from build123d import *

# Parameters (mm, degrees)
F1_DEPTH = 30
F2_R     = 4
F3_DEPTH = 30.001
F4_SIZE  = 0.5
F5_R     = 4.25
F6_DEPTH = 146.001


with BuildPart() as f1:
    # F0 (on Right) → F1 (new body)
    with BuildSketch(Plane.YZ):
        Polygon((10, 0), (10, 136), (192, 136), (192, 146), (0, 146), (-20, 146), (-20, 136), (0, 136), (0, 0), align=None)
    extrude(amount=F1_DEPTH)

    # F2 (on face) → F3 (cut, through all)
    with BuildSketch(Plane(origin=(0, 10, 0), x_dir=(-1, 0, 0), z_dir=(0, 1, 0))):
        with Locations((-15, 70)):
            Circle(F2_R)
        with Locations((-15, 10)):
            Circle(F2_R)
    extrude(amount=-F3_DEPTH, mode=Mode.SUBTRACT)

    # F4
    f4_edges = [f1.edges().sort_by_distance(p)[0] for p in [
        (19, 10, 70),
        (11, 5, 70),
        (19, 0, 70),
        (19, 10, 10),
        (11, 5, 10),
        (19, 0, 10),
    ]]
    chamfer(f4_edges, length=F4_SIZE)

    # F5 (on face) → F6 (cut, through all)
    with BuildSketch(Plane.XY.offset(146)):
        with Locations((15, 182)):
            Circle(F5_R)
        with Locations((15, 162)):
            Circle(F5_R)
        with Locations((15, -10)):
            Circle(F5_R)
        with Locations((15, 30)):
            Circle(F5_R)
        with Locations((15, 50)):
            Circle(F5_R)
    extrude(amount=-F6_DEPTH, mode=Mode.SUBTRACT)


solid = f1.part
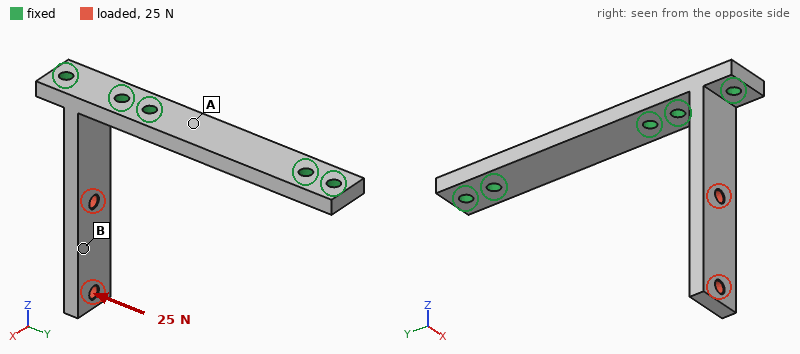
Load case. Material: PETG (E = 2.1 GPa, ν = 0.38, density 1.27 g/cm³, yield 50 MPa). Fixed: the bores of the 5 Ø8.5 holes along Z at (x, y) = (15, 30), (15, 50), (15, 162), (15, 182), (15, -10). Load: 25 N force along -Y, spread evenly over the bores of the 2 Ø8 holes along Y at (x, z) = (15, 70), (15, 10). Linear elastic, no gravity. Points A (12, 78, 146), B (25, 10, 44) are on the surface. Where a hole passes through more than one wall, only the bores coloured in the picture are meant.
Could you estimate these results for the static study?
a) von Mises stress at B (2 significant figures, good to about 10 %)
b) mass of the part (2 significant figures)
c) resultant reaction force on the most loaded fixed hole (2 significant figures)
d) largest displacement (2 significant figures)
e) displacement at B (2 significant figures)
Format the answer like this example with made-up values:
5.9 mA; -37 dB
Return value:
0.85 MPa; 130 g; 88 N; 2.7 mm; 1.5 mm
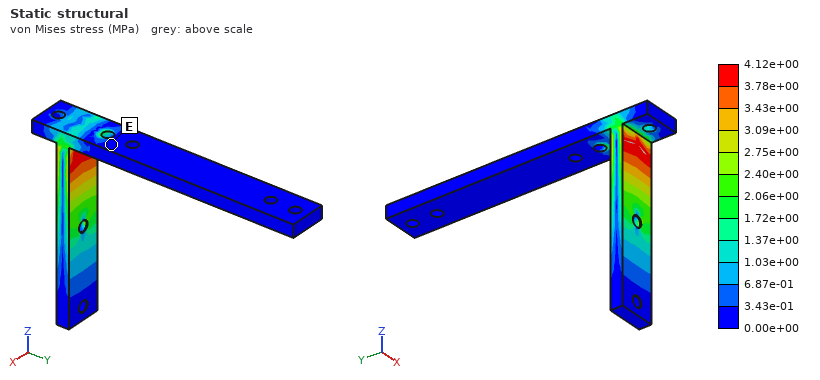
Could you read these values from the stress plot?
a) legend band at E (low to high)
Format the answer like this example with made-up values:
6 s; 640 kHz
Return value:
0.00e+00 to 3.43e-01 MPa
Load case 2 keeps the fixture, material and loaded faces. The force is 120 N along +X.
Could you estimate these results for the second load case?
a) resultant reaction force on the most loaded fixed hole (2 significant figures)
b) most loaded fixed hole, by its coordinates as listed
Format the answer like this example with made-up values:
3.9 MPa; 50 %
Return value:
82 N; (15, -10)
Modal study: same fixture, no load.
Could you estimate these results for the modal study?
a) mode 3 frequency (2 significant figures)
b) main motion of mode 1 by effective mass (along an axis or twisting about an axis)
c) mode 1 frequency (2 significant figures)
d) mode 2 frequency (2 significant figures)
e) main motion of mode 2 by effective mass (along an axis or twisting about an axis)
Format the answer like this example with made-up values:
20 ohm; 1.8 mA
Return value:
650 Hz; along Y; 110 Hz; 220 Hz; along X
